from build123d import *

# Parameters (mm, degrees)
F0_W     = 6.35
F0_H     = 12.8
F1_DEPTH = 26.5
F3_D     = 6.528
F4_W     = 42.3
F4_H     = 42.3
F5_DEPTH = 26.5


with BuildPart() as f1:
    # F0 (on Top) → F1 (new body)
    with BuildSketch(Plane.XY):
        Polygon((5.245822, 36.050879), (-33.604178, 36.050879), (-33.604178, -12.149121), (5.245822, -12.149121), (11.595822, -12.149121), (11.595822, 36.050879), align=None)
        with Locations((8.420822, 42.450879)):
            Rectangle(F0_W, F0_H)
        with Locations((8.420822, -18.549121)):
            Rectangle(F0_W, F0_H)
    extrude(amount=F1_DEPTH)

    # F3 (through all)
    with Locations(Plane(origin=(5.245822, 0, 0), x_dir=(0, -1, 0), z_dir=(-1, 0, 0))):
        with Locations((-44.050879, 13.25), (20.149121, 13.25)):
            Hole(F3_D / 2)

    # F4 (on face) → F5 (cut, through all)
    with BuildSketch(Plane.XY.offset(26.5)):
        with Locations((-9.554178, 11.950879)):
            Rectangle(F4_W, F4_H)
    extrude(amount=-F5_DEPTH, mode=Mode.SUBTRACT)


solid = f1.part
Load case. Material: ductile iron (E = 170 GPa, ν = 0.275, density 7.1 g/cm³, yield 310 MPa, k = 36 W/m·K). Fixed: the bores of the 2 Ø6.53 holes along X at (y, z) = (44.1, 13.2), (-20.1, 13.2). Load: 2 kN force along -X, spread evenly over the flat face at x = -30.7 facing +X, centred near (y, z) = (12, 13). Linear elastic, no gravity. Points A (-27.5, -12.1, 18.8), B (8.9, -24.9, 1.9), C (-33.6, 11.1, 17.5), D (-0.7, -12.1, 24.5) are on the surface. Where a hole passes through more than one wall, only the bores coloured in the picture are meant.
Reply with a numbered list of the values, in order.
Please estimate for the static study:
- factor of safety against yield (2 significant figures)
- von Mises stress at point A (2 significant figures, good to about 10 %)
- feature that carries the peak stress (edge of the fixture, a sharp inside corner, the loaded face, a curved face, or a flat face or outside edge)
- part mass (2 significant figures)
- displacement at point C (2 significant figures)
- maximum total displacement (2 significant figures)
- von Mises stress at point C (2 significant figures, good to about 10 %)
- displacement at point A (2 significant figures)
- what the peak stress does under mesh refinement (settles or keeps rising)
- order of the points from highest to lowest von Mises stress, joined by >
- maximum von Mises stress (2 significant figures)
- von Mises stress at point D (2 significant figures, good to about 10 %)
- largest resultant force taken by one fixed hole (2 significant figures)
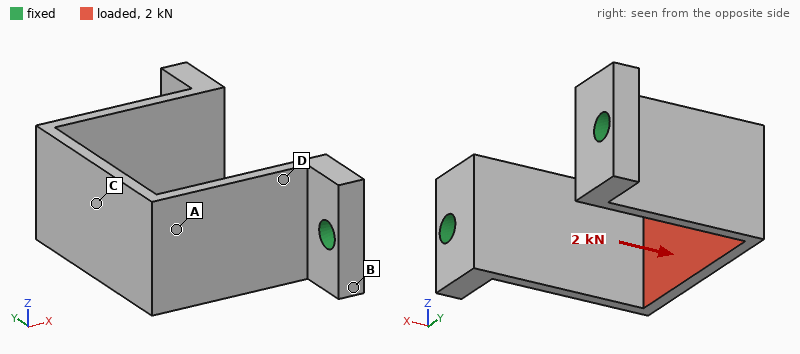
1. 1.8
2. 100 MPa
3. a flat face or outside edge
4. 100 g
5. 0.12 mm
6. 0.12 mm
7. 160 MPa
8. 0.020 mm
9. settles
10. C > A > D > B
11. 170 MPa
12. 47 MPa
13. 1.0 kN
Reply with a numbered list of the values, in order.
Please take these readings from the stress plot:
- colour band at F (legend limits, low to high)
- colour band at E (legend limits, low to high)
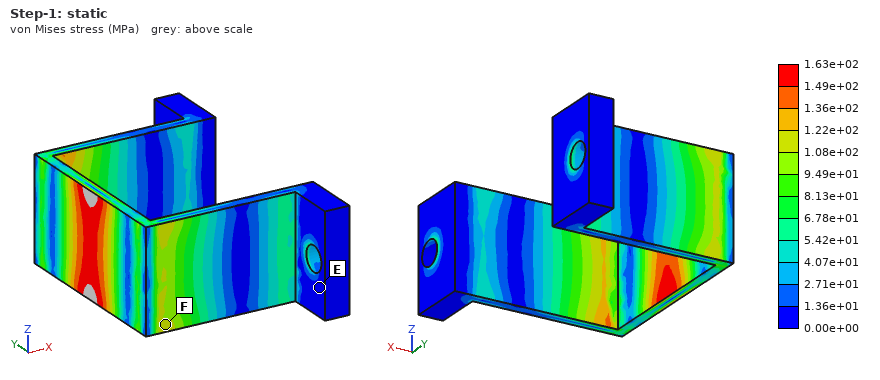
1. 1.08e+02 to 1.22e+02 MPa
2. 0.00e+00 to 1.36e+01 MPa
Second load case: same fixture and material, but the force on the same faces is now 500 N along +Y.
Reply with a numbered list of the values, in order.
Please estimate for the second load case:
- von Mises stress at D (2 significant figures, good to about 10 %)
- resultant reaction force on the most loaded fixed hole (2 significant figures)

1. 95 MPa
2. 300 N
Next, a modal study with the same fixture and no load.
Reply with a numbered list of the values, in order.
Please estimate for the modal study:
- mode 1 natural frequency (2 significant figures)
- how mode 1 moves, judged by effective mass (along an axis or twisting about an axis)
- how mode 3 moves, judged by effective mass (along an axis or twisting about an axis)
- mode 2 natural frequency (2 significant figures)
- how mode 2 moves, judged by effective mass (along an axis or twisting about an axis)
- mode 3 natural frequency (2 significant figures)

1. 1300 Hz
2. along Y
3. twisting about X
4. 2900 Hz
5. along Z
6. 3700 Hz
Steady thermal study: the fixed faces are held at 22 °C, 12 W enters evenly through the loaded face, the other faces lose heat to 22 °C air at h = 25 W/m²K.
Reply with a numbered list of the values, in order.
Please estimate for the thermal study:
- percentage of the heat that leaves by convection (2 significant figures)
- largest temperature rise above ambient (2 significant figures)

1. 50 %
2. 74 K
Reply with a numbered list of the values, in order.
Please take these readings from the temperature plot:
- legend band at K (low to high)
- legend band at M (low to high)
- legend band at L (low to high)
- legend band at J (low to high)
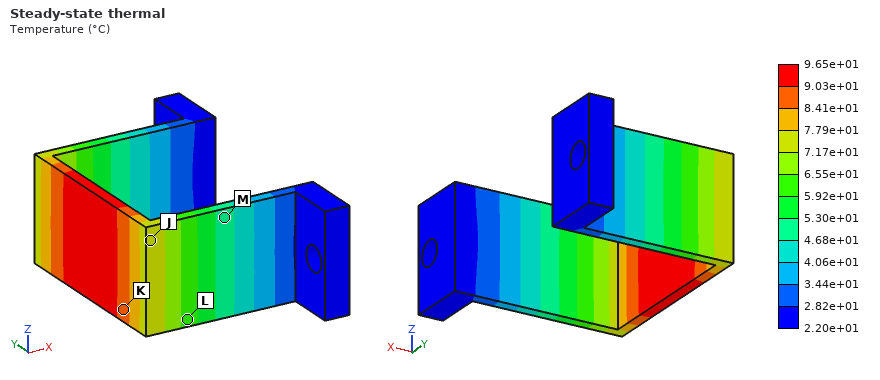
1. 8.41e+01 to 9.03e+01 °C
2. 4.68e+01 to 5.30e+01 °C
3. 5.92e+01 to 6.55e+01 °C
4. 7.17e+01 to 7.79e+01 °C
